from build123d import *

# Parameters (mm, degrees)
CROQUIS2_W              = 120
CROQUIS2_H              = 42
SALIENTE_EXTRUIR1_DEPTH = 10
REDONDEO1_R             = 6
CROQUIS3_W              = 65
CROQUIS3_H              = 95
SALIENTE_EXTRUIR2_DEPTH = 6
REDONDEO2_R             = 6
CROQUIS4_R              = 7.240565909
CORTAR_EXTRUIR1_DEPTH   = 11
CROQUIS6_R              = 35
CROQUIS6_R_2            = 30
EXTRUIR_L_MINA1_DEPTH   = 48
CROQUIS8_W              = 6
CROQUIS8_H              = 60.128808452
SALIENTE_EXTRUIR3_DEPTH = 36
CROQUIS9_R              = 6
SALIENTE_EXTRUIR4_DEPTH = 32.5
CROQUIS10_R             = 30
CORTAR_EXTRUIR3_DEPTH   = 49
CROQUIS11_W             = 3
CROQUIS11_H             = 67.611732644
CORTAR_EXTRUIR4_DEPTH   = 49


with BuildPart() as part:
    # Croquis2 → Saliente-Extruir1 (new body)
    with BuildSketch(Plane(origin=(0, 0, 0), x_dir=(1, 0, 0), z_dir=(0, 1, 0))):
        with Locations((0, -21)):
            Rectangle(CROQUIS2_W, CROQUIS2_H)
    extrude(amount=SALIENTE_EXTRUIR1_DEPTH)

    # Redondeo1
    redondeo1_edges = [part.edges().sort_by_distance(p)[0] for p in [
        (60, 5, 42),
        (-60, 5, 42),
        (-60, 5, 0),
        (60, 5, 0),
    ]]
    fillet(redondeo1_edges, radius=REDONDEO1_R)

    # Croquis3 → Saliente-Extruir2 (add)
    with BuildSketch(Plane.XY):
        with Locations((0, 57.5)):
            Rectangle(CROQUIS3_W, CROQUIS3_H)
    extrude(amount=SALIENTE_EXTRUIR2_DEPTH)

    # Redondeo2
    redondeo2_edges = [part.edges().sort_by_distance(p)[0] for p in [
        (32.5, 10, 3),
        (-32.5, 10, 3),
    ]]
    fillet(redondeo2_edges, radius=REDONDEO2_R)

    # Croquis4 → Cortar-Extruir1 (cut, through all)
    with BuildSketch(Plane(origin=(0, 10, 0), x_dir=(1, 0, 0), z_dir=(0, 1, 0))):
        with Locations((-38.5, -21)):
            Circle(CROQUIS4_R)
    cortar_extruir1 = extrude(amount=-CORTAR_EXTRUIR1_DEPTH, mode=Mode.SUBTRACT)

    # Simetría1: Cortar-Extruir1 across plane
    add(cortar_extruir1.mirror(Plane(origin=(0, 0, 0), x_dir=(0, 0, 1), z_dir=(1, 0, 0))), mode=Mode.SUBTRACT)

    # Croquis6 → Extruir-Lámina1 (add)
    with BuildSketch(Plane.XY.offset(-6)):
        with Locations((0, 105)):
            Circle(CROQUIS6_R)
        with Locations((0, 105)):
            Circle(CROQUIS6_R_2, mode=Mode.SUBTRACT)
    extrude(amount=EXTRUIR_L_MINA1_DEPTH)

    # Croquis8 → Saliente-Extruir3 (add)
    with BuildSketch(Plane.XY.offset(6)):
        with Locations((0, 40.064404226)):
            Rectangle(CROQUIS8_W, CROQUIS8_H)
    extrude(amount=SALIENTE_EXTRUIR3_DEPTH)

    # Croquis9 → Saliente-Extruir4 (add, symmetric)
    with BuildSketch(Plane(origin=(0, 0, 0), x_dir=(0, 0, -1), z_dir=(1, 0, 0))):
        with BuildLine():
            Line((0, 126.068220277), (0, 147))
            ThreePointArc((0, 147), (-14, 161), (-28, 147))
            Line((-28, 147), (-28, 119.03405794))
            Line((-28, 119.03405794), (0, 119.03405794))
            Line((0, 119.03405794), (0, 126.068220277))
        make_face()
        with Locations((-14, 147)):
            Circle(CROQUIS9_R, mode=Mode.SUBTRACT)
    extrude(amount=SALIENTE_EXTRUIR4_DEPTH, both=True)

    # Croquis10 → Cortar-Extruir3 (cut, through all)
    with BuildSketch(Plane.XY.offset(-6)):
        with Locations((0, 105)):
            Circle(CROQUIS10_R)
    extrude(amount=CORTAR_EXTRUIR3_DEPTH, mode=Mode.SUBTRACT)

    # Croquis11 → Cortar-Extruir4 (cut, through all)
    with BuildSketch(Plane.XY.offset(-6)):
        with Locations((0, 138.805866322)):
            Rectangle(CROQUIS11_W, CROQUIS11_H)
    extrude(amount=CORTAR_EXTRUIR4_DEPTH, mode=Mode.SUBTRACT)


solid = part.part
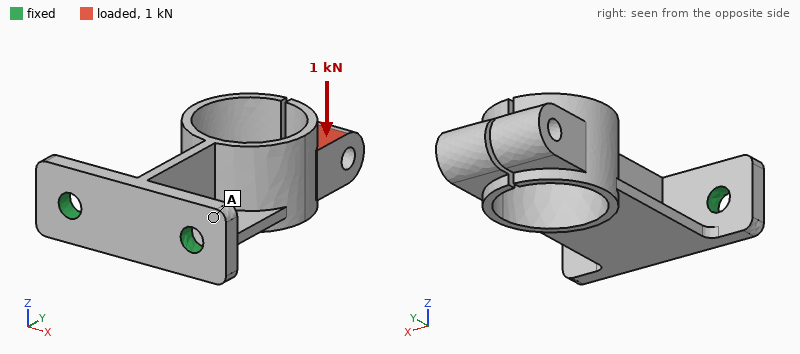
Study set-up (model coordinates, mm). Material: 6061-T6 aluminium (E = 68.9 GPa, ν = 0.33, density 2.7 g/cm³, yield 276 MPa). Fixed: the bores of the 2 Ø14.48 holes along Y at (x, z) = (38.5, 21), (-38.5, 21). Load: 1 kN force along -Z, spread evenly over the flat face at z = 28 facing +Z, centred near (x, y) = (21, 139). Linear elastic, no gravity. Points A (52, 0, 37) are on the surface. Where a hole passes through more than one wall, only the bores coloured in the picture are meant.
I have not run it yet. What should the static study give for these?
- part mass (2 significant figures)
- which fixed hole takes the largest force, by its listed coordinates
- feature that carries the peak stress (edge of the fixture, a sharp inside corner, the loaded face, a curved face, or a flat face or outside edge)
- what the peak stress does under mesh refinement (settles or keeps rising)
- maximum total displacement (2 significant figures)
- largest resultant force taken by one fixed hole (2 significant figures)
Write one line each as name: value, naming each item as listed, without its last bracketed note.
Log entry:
part mass: 460 g
which fixed hole takes the largest force, by its listed coordinates: (38.5, 21)
feature that carries the peak stress: a sharp inside corner
what the peak stress does under mesh refinement: keeps rising
maximum total displacement: 2.1 mm
largest resultant force taken by one fixed hole: 840 N
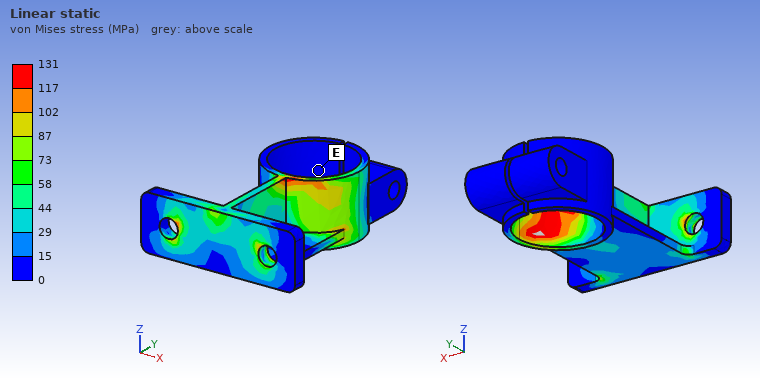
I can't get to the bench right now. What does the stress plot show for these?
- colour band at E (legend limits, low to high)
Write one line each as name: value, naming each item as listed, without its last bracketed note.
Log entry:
colour band at E: 0 to 15 MPa
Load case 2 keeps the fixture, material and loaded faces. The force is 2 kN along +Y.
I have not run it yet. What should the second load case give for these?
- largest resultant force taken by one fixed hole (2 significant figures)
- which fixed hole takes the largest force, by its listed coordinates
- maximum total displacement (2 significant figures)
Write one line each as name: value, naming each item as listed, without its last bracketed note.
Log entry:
largest resultant force taken by one fixed hole: 1.6 kN
which fixed hole takes the largest force, by its listed coordinates: (38.5, 21)
maximum total displacement: 1.4 mm
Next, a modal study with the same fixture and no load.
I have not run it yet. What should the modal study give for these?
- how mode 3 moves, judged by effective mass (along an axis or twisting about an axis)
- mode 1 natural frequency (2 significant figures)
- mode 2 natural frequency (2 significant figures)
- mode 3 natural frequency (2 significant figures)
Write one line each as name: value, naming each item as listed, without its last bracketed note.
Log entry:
how mode 3 moves, judged by effective mass: along Z
mode 1 natural frequency: 350 Hz
mode 2 natural frequency: 350 Hz
mode 3 natural frequency: 440 Hz
